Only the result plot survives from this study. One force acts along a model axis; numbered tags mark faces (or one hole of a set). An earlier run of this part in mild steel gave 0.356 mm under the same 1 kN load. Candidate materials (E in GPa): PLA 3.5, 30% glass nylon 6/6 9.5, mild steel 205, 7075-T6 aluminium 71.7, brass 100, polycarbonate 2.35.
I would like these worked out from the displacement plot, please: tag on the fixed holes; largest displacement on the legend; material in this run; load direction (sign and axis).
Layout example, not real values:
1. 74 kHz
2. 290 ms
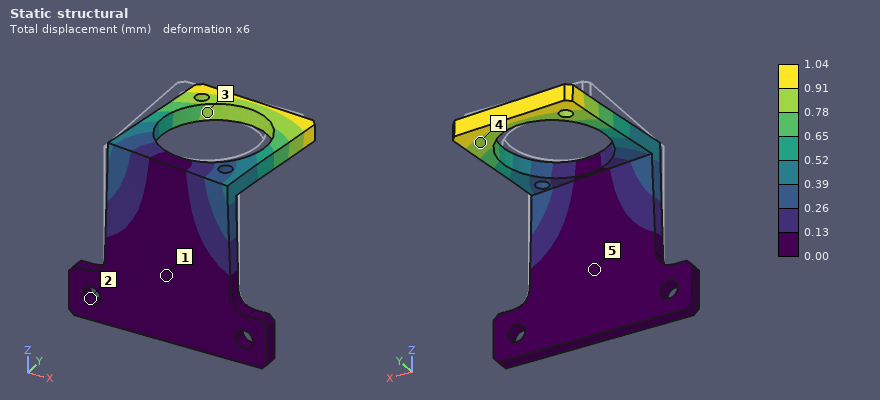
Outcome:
1. 2
2. 1.04 mm
3. 7075-T6 aluminium
4. +X
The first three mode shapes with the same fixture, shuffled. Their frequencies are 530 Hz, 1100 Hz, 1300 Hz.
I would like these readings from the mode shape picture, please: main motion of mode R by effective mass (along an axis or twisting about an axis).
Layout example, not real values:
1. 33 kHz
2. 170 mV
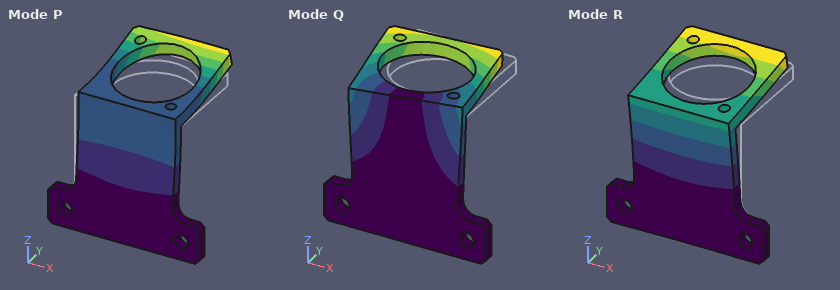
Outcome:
1. along Y
